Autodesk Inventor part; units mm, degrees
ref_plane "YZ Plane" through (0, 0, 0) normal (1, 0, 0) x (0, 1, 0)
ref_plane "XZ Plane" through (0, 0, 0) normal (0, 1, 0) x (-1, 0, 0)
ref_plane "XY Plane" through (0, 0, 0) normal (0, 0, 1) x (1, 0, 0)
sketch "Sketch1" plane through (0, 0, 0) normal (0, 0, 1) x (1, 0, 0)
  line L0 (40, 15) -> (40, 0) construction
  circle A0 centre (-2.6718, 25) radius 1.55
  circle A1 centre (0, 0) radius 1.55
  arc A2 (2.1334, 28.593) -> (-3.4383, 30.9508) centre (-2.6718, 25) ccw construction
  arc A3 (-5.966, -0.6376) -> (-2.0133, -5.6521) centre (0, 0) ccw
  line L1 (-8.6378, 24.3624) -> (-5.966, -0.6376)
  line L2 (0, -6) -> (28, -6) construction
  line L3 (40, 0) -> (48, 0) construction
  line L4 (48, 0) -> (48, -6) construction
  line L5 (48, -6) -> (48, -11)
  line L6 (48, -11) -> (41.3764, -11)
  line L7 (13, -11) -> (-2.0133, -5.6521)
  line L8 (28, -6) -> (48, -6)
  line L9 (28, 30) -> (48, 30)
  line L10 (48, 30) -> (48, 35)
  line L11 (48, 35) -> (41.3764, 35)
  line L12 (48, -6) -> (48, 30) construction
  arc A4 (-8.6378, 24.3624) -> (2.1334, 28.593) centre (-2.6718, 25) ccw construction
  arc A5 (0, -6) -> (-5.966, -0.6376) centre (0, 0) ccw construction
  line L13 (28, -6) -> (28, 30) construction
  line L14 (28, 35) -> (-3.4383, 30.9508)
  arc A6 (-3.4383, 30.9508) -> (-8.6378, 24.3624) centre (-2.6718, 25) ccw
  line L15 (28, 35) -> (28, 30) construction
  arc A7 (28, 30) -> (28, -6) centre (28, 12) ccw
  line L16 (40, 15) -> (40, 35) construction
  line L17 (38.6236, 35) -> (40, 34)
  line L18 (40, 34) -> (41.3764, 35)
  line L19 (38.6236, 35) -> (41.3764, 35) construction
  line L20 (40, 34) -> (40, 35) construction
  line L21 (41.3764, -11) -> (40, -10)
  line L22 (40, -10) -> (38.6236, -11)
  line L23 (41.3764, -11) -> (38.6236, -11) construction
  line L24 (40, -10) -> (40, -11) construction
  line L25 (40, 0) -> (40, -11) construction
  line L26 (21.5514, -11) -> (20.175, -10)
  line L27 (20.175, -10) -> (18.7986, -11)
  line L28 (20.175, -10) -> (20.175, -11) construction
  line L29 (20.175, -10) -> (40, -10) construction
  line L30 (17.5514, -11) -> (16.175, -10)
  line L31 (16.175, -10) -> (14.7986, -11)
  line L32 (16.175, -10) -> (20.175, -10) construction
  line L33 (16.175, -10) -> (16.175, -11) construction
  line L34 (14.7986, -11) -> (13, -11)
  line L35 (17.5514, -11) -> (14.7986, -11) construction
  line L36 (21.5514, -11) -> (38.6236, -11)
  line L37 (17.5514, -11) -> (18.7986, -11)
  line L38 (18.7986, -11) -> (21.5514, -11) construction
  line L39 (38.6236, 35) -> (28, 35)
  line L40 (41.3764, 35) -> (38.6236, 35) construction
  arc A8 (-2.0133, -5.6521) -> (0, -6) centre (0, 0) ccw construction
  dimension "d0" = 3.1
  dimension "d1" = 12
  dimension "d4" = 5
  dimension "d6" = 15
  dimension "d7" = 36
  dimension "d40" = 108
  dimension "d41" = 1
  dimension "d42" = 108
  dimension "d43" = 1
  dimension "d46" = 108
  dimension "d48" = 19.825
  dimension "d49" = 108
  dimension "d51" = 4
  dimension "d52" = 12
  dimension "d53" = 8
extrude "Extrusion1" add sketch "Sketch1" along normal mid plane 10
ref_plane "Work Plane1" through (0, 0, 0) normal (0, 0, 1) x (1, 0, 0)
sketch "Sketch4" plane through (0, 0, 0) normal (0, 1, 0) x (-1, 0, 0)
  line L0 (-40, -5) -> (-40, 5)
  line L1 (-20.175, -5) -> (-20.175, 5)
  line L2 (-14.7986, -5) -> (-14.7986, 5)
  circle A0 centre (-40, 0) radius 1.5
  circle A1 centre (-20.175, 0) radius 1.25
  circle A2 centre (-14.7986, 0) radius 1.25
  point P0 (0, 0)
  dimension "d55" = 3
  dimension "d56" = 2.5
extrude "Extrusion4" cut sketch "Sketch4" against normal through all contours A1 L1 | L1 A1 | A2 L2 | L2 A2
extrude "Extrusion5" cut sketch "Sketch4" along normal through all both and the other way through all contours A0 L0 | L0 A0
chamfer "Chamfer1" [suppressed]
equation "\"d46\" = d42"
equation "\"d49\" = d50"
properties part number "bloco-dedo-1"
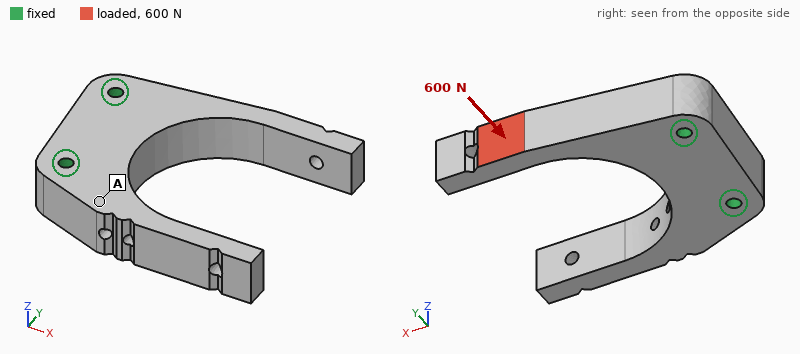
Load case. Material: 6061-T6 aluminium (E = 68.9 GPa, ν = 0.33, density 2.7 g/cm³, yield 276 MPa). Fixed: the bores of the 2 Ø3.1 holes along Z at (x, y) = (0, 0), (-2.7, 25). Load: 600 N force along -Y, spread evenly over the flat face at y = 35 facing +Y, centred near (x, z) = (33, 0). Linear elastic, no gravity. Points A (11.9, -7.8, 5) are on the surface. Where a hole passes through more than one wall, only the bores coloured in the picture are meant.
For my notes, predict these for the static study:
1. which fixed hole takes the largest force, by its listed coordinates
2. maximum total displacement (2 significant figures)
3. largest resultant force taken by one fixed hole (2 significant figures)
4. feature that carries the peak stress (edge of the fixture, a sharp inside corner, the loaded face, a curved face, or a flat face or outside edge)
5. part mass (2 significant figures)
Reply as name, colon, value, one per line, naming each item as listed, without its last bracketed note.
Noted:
which fixed hole takes the largest force, by its listed coordinates: (0, 0)
maximum total displacement: 0.39 mm
largest resultant force taken by one fixed hole: 1.1 kN
feature that carries the peak stress: a curved face
part mass: 30 g
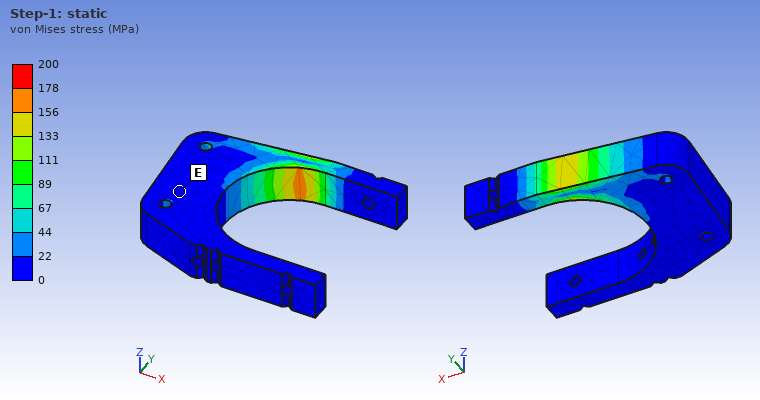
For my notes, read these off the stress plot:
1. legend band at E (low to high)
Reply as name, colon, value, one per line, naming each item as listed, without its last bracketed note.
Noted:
legend band at E: 0 to 22 MPa
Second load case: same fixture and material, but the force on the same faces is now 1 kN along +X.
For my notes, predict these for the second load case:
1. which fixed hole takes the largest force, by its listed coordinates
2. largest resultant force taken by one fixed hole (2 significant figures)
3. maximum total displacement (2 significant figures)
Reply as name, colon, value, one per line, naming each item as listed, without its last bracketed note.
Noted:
which fixed hole takes the largest force, by its listed coordinates: (-2.7, 25)
largest resultant force taken by one fixed hole: 1.4 kN
maximum total displacement: 0.22 mm
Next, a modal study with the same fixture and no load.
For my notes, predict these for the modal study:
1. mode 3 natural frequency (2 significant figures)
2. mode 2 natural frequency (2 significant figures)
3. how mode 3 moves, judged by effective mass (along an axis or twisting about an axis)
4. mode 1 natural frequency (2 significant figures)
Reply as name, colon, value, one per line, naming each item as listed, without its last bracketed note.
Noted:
mode 3 natural frequency: 4300 Hz
mode 2 natural frequency: 4000 Hz
how mode 3 moves, judged by effective mass: along Z
mode 1 natural frequency: 3800 Hz
